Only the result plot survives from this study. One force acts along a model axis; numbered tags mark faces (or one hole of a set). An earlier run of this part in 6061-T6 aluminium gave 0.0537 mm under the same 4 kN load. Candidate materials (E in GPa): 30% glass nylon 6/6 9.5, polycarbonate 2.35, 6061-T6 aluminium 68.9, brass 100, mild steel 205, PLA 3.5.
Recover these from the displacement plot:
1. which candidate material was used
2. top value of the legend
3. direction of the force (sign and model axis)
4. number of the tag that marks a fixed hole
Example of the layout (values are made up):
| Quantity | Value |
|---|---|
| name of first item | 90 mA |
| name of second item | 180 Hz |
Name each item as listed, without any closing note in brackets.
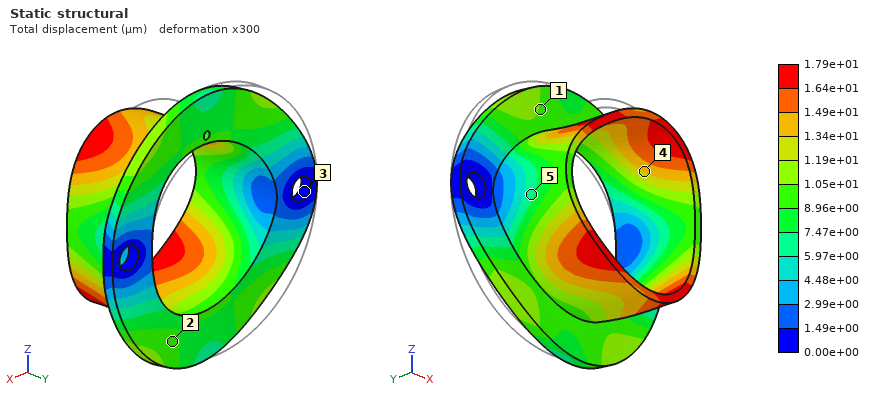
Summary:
| Quantity | Value |
|---|---|
| which candidate material was used | mild steel |
| top value of the legend | 1.79e+01 µm |
| direction of the force | +X |
| number of the tag that marks a fixed hole | 3 |
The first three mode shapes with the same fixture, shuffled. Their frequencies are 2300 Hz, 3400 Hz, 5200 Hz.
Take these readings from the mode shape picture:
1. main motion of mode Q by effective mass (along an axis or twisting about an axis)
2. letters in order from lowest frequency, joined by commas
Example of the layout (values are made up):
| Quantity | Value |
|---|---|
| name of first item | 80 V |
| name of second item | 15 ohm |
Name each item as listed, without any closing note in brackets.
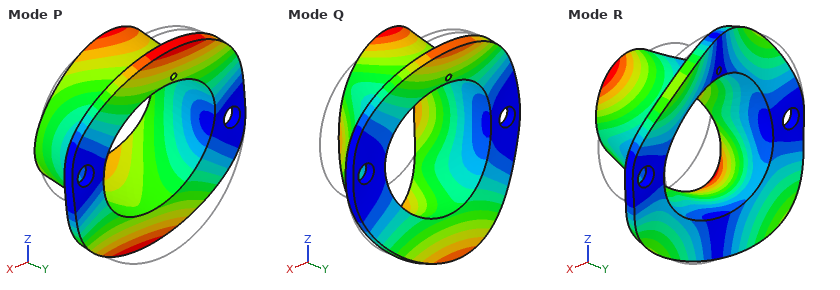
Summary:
| Quantity | Value |
|---|---|
| main motion of mode Q by effective mass | along Y |
| letters in order from lowest frequency, joined by commas | P, Q, R |
